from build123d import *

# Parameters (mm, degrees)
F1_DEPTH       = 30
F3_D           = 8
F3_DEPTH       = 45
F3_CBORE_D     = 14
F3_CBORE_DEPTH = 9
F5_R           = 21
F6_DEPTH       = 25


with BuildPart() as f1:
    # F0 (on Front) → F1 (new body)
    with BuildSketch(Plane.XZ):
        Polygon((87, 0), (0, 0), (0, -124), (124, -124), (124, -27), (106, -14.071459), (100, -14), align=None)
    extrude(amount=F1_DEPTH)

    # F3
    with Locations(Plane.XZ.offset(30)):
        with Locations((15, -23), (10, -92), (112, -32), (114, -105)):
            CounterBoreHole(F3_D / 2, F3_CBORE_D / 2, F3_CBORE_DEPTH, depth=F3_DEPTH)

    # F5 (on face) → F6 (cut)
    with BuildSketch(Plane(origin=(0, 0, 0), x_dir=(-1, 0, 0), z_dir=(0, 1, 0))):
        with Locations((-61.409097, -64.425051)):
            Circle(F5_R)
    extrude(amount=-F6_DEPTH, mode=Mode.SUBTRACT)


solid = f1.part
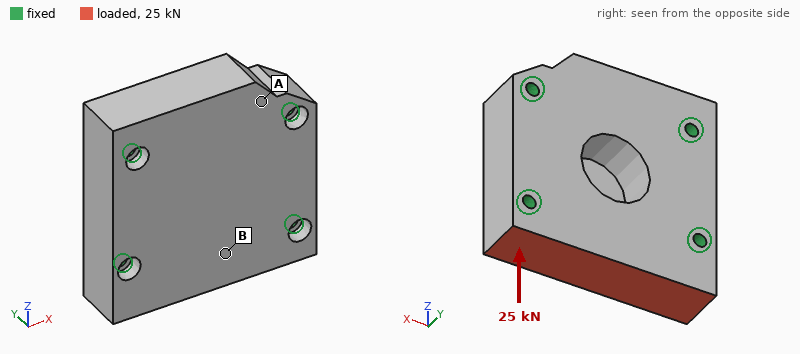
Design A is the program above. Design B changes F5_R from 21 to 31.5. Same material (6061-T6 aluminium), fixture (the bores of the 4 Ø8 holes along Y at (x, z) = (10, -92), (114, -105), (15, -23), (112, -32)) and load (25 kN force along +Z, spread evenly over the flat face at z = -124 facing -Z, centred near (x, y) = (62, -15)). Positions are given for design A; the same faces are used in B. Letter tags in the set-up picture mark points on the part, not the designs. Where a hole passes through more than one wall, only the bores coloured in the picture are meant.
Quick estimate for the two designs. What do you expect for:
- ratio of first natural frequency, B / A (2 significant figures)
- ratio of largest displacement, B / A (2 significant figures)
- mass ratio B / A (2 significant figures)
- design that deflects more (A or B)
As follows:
1.0
1.3
0.89
B
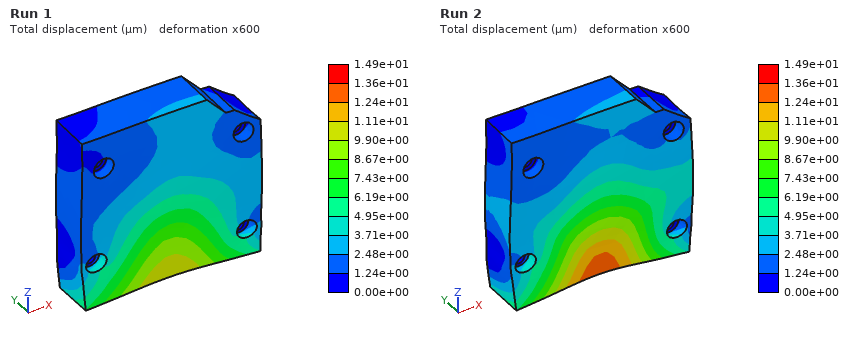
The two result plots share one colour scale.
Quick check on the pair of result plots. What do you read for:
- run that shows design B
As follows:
Run 2
